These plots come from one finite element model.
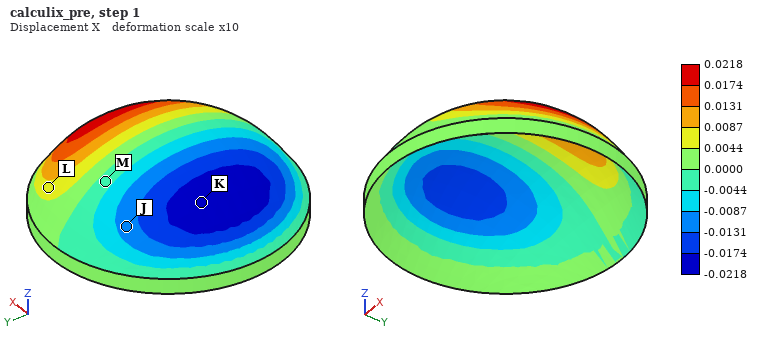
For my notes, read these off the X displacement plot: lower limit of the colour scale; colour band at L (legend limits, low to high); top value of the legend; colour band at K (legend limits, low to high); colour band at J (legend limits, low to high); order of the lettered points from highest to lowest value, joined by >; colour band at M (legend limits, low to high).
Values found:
-0.0218
0.0044 to 0.0087
0.0218
-0.0218 to -0.0174
-0.0131 to -0.0087
L > M > J > K
-0.0044 to 0.0000
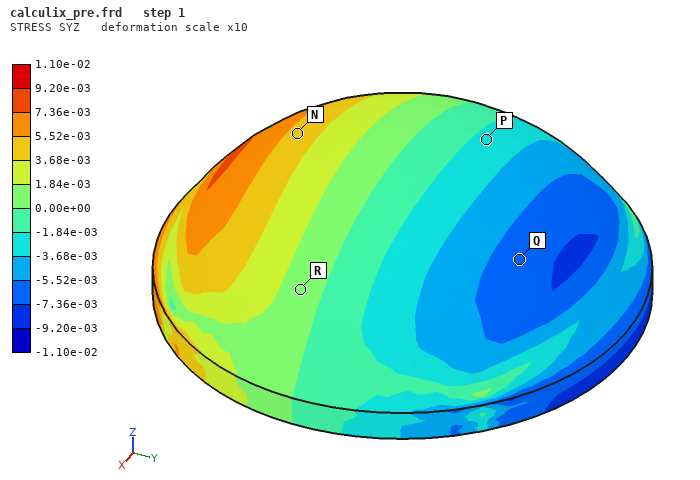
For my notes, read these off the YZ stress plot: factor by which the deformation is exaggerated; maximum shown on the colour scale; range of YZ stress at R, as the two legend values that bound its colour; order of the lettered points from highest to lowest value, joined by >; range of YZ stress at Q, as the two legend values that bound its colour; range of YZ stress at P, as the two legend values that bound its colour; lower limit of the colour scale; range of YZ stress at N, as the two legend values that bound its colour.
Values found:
10
1.10e-02
0.00e+00 to 1.84e-03
N > R > P > Q
-7.36e-03 to -5.52e-03
-3.68e-03 to -1.84e-03
-1.10e-02
3.68e-03 to 5.52e-03
